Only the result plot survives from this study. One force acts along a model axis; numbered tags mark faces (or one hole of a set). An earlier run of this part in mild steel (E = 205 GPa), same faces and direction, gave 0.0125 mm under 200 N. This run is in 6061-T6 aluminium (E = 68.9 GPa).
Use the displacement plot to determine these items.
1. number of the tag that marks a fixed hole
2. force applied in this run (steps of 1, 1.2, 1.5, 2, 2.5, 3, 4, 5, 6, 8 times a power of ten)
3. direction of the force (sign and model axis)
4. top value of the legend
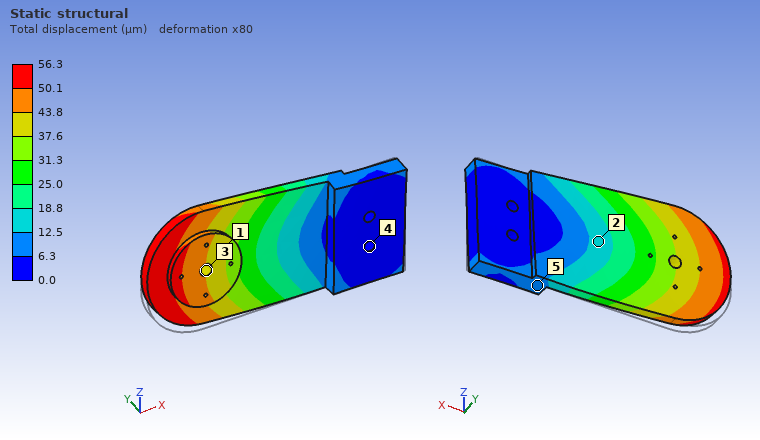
4
300 N
+Z
56.3 µm
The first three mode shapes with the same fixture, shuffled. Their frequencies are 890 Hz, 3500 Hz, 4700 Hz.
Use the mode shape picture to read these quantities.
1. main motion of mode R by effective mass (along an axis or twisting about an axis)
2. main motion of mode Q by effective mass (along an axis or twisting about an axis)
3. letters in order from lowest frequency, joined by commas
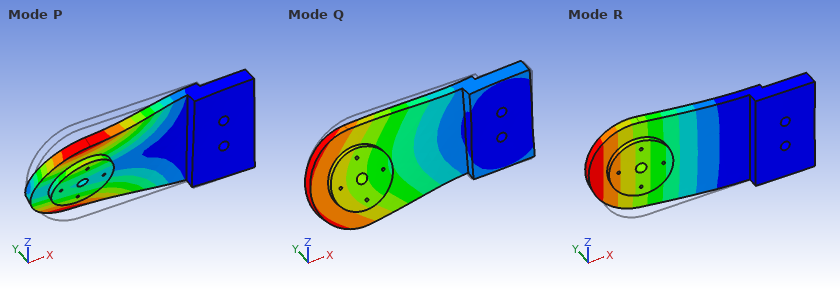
along Y
along Z
R, P, Q
